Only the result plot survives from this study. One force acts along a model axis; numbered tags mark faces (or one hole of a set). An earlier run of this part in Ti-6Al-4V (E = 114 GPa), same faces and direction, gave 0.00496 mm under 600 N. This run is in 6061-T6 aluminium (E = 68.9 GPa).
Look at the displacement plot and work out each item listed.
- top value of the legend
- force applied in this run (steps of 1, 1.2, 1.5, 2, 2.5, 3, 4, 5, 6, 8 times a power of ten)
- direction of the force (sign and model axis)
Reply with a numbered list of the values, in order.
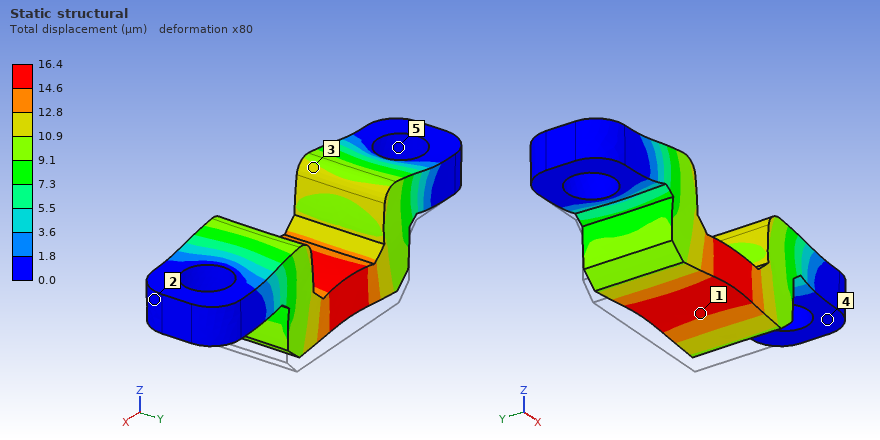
1. 16.4 µm
2. 1.2 kN
3. +Z
